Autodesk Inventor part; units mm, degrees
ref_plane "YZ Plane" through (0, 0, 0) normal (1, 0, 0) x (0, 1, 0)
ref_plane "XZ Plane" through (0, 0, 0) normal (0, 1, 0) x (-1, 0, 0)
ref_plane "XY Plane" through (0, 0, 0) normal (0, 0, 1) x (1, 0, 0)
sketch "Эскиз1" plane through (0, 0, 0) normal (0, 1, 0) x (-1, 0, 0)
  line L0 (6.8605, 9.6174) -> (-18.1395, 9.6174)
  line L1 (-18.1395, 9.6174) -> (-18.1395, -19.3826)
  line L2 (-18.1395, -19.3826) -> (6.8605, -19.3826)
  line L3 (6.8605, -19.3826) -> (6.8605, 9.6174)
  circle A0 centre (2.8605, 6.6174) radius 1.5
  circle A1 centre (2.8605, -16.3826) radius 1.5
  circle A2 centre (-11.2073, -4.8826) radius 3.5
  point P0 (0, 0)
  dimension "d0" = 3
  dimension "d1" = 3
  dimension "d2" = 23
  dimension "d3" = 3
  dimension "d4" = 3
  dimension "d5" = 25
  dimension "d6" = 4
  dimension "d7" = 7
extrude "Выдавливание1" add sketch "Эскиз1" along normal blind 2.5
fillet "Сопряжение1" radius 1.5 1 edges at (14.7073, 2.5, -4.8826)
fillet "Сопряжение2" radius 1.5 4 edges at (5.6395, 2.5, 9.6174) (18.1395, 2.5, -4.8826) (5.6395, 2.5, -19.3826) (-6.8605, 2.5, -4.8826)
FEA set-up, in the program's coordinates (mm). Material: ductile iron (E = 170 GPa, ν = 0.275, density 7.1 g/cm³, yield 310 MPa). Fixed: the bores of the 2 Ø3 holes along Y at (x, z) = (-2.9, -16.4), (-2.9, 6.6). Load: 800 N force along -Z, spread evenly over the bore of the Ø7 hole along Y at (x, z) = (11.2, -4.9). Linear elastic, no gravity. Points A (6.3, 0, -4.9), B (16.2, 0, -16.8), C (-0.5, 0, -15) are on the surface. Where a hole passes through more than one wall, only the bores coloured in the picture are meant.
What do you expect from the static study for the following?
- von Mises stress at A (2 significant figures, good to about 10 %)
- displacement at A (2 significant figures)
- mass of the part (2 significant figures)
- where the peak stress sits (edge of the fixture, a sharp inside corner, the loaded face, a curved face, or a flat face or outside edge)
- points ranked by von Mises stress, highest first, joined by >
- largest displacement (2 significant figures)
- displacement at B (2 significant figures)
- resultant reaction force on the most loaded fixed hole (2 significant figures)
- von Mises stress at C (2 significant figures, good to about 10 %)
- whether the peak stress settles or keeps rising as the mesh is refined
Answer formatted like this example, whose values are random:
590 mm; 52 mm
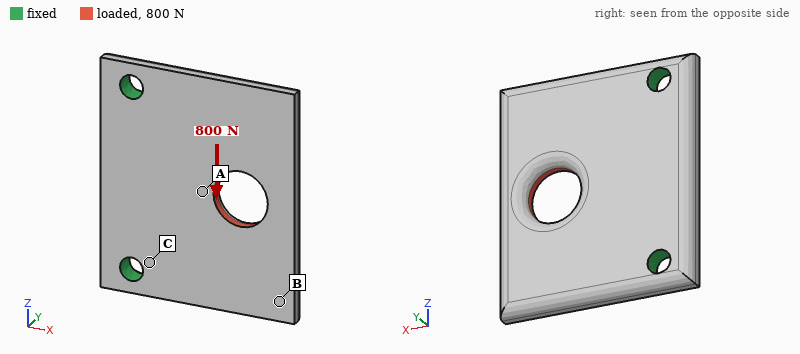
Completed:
55 MPa; 2.8 µm; 11 g; edge of the fixture; A > C > B; 11 µm; 8.9 µm; 610 N; 33 MPa; keeps rising
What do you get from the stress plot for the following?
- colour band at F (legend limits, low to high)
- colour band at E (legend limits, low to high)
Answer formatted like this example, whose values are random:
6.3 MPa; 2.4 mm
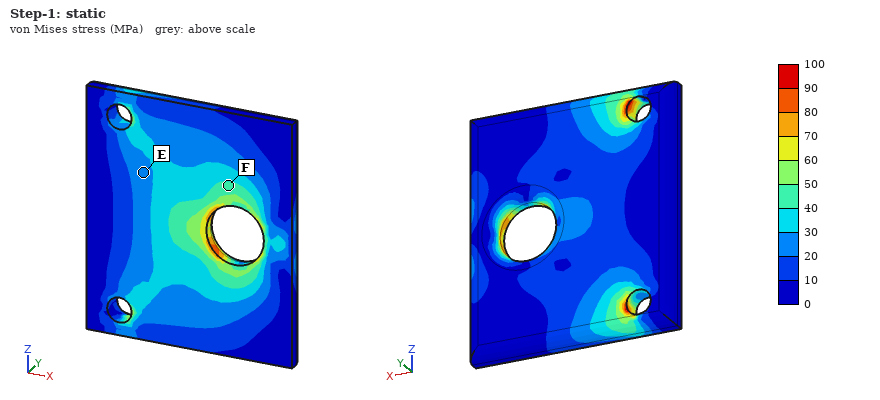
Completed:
40 to 50 MPa; 20 to 30 MPa
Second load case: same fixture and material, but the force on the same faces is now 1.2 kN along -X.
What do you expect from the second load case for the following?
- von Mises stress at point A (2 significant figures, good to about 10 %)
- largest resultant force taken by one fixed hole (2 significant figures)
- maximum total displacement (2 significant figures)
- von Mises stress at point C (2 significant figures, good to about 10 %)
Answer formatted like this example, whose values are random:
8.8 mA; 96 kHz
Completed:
57 MPa; 630 N; 35 µm; 87 MPa
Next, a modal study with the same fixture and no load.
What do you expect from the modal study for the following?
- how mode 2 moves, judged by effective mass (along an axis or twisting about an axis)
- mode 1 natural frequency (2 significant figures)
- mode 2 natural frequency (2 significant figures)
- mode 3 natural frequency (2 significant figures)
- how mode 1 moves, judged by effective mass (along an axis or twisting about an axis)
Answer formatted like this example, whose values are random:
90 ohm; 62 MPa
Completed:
twisting about X; 4300 Hz; 8500 Hz; 18 kHz; along Y
